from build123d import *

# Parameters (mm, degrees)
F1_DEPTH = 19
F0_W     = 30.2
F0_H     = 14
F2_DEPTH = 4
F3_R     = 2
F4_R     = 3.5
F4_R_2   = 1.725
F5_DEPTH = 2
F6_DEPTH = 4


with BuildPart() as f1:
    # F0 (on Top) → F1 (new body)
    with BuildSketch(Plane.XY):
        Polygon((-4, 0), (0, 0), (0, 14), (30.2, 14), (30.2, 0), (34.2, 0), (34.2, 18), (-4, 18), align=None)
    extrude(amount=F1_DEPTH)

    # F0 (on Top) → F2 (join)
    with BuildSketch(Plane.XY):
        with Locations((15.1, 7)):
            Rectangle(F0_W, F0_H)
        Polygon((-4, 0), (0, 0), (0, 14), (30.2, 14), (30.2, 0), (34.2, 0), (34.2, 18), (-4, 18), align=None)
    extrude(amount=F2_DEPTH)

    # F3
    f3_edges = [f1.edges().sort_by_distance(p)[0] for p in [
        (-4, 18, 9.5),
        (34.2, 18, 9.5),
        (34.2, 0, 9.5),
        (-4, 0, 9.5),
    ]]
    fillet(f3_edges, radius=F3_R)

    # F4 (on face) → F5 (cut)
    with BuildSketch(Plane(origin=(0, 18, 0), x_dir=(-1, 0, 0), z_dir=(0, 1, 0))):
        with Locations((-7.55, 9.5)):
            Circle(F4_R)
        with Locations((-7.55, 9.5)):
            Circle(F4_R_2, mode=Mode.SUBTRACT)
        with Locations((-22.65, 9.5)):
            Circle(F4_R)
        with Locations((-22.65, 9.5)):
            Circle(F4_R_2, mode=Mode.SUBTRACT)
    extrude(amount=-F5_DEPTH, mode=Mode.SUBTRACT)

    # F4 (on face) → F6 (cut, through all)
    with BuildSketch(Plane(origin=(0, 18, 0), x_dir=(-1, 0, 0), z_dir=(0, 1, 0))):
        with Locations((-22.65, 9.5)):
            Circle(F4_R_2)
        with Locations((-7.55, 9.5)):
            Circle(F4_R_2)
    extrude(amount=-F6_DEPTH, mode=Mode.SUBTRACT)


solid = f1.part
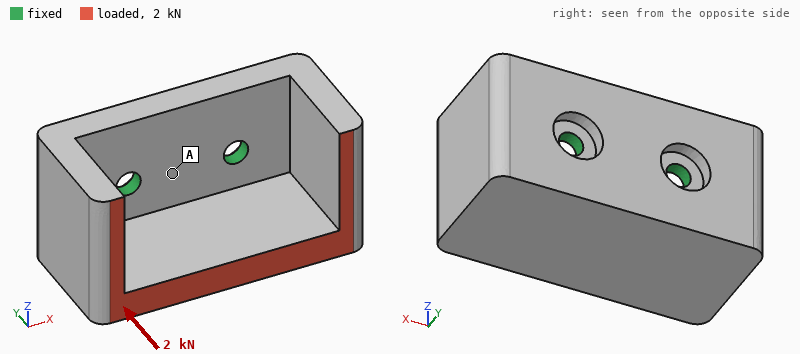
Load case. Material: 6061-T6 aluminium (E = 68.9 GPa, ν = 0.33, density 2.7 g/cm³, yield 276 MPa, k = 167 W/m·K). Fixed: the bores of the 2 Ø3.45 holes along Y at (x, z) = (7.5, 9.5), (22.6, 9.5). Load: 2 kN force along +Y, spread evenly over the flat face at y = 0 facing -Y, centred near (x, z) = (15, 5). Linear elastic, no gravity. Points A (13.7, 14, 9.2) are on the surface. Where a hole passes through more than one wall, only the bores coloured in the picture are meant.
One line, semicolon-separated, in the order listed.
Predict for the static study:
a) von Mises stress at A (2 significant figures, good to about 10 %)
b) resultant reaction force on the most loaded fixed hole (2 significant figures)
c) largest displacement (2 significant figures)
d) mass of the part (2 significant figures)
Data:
41 MPa; 1.0 kN; 0.11 mm; 17 g
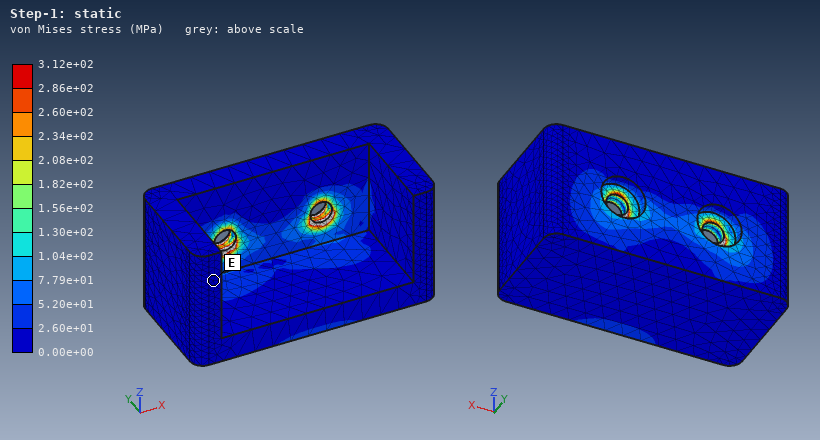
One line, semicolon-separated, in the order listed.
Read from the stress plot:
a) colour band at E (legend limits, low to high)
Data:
0.00e+00 to 2.60e+01 MPa
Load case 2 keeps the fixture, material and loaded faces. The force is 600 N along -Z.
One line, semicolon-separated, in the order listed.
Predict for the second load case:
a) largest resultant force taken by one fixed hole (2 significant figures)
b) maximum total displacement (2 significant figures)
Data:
350 N; 0.14 mm
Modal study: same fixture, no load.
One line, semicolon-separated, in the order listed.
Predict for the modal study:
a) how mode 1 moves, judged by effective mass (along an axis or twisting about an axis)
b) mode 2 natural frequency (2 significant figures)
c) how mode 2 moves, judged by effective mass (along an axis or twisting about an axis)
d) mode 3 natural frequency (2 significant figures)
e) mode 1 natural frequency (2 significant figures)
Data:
along Z; 7000 Hz; along X; 10 kHz; 4800 Hz
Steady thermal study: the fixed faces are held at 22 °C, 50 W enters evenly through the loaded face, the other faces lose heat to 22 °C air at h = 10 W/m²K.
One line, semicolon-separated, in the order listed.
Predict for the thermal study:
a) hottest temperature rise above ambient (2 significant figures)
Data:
39 K
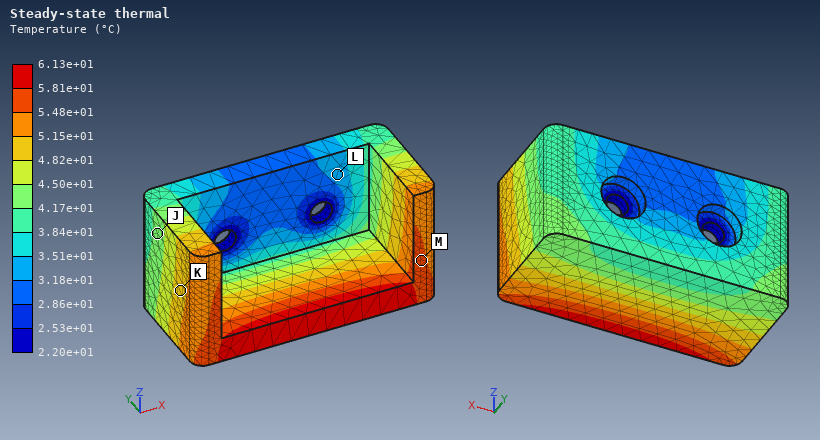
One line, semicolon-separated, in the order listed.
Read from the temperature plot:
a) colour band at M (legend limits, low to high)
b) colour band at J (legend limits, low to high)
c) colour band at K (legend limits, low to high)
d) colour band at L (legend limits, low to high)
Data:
5.48e+01 to 5.81e+01 °C; 4.17e+01 to 4.50e+01 °C; 4.82e+01 to 5.15e+01 °C; 3.18e+01 to 3.51e+01 °C
